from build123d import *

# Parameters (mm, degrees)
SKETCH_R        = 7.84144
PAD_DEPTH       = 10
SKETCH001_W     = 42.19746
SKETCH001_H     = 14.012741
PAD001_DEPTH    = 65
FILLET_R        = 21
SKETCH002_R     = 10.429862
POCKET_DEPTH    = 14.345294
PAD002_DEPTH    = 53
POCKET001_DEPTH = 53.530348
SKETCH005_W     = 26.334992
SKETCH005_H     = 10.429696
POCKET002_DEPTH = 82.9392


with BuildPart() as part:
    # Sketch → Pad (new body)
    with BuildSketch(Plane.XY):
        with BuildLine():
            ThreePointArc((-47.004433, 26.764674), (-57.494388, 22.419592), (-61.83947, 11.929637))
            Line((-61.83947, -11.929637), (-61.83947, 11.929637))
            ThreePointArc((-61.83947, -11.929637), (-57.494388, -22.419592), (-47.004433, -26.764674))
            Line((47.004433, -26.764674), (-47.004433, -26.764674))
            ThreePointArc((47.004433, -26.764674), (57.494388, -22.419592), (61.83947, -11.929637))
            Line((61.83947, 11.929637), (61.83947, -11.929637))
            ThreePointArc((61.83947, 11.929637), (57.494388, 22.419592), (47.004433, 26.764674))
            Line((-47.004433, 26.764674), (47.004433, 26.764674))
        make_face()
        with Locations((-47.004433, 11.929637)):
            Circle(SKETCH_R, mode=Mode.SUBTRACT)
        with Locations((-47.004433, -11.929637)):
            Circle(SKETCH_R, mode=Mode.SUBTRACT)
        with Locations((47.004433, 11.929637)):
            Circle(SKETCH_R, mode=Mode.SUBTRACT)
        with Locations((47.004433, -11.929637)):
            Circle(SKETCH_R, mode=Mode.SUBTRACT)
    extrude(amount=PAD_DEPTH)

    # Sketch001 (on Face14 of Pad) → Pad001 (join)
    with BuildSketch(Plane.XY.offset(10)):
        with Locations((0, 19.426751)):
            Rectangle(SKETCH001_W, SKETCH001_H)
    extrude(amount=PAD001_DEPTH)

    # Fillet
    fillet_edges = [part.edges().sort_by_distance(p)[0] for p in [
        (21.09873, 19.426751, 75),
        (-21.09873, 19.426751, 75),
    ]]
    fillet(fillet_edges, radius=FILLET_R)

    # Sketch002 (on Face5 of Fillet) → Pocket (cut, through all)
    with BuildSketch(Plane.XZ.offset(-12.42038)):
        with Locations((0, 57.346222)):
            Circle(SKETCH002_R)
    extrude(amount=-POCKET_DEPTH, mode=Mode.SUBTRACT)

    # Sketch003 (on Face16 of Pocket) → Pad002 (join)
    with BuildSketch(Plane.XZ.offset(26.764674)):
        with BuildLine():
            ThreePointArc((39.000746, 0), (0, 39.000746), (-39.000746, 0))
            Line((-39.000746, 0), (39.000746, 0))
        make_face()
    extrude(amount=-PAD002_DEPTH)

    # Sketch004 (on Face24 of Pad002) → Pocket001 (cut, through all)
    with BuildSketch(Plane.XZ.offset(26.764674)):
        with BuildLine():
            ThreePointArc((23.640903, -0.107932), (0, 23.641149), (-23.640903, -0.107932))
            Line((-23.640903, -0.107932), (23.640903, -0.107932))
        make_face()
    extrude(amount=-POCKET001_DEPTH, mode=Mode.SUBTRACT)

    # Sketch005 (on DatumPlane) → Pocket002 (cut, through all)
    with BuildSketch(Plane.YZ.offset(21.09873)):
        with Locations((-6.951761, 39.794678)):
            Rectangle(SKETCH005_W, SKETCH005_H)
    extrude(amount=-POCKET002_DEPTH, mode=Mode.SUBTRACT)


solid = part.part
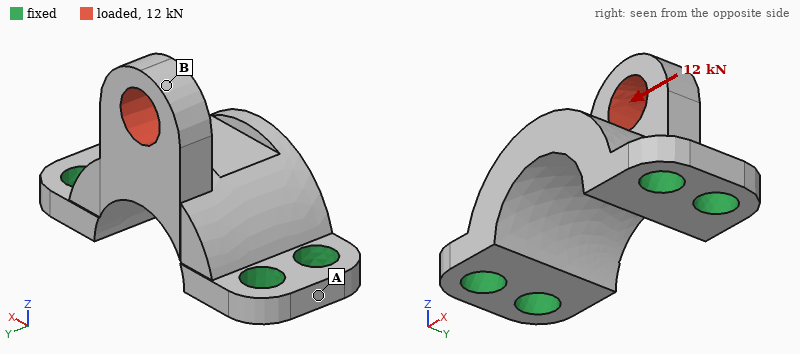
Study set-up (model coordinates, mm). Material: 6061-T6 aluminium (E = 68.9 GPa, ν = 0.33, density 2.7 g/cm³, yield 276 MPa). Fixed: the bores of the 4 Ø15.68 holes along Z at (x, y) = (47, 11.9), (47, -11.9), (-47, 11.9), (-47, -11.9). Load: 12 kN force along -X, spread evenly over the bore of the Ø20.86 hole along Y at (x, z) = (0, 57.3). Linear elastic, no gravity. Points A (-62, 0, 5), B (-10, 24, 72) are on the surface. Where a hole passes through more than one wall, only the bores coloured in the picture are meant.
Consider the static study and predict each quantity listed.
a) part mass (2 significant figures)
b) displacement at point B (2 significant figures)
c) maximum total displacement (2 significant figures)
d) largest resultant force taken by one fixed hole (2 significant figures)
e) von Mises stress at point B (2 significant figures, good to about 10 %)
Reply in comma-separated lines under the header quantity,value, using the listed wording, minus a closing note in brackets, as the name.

quantity,value
part mass,290 g
displacement at point B,0.15 mm
maximum total displacement,0.15 mm
largest resultant force taken by one fixed hole,6.7 kN
von Mises stress at point B,54 MPa
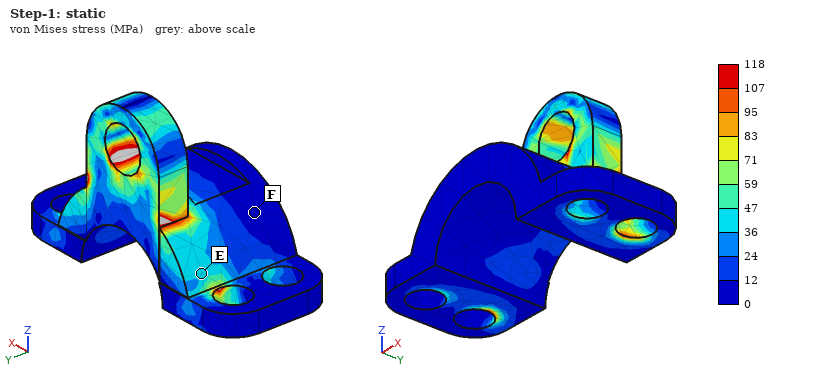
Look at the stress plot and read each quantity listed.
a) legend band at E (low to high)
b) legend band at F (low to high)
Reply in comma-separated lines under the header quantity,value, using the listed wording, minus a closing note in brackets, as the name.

quantity,value
legend band at E,36 to 47 MPa
legend band at F,0 to 12 MPa
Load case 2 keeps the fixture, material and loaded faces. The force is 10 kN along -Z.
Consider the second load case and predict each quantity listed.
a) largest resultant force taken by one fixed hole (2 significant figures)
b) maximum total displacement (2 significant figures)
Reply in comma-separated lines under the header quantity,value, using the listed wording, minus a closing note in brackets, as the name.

quantity,value
largest resultant force taken by one fixed hole,6.7 kN
maximum total displacement,79 µm
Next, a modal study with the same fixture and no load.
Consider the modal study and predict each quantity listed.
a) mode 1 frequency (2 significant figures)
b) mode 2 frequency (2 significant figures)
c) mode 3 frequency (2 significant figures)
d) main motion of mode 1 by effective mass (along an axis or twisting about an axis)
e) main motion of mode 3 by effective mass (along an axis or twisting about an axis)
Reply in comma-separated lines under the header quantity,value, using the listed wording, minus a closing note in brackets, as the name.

quantity,value
mode 1 frequency,4700 Hz
mode 2 frequency,8600 Hz
mode 3 frequency,9400 Hz
main motion of mode 1 by effective mass,along Y
main motion of mode 3 by effective mass,along Y
